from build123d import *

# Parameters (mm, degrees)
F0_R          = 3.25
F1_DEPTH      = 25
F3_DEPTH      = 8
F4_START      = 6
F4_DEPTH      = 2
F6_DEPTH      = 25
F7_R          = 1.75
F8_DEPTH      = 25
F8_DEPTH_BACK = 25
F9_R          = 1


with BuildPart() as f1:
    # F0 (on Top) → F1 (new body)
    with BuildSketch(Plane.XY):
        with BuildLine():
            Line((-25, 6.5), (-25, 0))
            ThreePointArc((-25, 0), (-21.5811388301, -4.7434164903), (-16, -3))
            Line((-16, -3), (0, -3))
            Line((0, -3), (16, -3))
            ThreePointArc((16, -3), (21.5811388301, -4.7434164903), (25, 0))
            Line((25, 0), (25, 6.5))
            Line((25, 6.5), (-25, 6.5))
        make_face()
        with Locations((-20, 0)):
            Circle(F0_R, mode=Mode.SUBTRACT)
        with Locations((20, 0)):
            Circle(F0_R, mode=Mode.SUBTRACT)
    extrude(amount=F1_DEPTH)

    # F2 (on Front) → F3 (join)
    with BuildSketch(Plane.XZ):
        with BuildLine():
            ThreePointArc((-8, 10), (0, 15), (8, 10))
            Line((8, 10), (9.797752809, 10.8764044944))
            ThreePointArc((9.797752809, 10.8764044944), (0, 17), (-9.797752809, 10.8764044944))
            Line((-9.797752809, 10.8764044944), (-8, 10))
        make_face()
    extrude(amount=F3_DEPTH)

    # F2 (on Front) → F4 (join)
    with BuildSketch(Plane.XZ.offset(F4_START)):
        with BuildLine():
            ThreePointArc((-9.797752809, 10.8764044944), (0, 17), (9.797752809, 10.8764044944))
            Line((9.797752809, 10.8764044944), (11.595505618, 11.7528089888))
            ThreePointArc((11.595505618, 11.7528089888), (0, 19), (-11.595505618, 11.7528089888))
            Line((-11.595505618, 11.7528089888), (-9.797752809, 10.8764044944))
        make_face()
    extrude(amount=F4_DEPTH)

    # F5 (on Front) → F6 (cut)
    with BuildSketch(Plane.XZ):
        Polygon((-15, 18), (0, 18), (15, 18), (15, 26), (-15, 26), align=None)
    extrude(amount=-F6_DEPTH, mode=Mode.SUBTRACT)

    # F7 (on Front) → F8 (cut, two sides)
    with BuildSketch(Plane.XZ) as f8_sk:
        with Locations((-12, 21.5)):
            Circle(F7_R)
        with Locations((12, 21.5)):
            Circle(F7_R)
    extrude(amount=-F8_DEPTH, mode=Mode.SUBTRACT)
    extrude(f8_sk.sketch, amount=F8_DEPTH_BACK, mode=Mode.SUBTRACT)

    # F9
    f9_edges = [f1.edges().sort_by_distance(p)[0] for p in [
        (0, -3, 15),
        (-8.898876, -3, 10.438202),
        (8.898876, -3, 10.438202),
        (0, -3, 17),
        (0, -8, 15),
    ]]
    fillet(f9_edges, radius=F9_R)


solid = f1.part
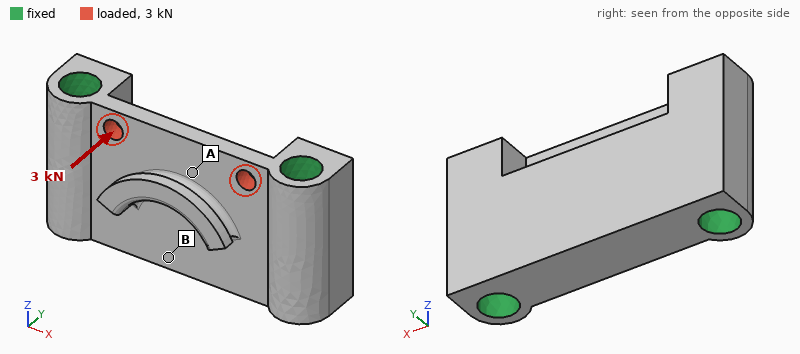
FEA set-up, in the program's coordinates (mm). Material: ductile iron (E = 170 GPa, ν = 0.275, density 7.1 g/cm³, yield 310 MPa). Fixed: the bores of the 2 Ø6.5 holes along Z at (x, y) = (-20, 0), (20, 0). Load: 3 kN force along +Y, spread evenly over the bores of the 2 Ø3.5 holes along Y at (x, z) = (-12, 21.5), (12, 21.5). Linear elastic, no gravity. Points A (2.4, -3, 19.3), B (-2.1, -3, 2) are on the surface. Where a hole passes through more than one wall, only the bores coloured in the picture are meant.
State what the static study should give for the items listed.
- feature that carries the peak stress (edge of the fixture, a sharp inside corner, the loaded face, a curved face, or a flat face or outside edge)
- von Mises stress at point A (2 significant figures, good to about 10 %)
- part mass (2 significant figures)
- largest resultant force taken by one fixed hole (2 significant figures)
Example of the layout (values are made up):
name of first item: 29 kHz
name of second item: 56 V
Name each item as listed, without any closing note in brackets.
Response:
feature that carries the peak stress: the loaded face
von Mises stress at point A: 33 MPa
part mass: 68 g
largest resultant force taken by one fixed hole: 1.5 kN
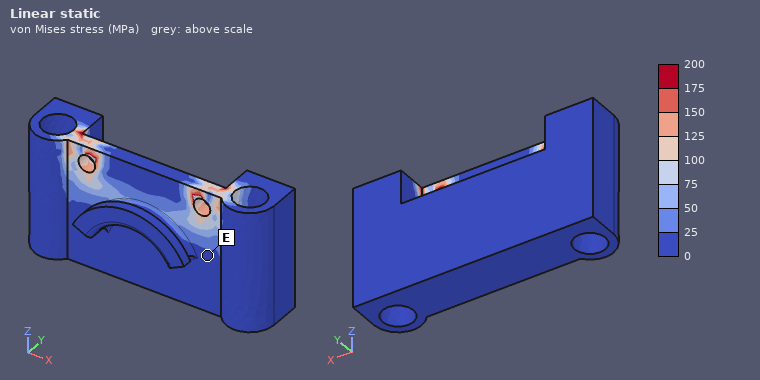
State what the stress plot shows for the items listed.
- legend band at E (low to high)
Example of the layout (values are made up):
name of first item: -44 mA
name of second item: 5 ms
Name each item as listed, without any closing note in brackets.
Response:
legend band at E: 0 to 25 MPa
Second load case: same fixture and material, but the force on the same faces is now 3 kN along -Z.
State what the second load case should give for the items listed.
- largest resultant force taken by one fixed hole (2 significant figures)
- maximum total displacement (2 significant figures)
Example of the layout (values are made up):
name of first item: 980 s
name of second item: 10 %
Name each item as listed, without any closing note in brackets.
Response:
largest resultant force taken by one fixed hole: 1.5 kN
maximum total displacement: 3.9 µm
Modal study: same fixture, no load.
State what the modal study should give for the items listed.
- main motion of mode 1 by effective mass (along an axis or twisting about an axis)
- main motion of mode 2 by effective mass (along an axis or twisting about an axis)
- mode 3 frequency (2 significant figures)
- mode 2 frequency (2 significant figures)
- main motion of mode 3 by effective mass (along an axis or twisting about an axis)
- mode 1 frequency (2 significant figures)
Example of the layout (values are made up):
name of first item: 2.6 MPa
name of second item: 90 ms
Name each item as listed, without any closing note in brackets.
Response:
main motion of mode 1 by effective mass: along Y
main motion of mode 2 by effective mass: along Y
mode 3 frequency: 35 kHz
mode 2 frequency: 29 kHz
main motion of mode 3 by effective mass: along Z
mode 1 frequency: 23 kHz
